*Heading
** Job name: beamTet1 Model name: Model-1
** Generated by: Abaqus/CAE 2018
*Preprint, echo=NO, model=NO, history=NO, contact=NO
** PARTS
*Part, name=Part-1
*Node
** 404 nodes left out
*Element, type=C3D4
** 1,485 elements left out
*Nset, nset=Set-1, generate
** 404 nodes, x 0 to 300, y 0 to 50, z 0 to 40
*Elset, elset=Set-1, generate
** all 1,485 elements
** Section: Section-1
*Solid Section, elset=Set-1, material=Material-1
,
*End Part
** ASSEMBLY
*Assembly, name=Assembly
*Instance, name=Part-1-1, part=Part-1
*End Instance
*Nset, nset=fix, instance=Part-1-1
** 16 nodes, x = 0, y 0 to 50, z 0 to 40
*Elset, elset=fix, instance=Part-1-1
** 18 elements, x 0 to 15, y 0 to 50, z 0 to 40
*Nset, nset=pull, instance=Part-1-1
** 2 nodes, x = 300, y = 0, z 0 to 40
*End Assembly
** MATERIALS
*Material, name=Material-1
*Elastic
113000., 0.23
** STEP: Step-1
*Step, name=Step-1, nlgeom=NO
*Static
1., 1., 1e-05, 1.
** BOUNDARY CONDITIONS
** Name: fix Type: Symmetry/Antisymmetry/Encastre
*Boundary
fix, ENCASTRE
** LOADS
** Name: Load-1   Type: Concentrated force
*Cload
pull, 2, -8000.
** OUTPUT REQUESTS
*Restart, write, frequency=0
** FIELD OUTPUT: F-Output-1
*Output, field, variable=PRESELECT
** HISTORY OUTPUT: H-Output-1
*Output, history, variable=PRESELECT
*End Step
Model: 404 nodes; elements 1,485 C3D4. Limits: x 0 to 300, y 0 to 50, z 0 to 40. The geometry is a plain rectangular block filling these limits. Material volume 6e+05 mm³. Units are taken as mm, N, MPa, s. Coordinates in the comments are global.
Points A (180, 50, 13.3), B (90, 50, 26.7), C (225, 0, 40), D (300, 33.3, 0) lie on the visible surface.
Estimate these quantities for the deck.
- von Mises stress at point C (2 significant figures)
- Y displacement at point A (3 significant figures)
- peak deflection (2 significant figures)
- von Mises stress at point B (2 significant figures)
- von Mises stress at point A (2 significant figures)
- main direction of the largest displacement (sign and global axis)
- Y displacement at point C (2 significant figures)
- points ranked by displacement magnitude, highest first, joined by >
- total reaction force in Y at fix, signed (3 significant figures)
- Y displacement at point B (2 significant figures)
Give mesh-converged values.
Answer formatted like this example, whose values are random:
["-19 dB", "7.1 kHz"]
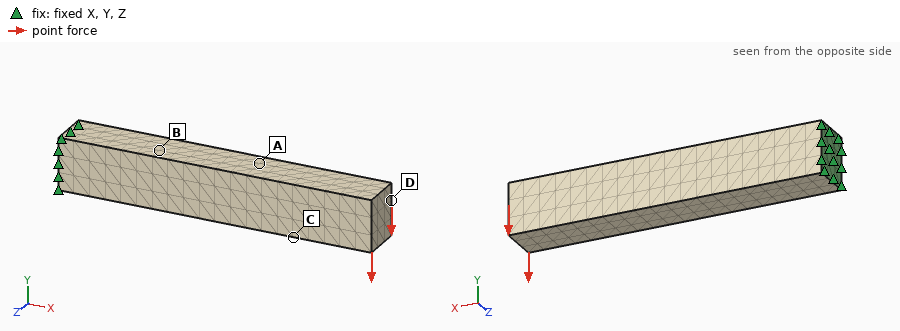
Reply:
["72 MPa", "-1.35 mm", "3.2 mm", "200 MPa", "120 MPa", "-Y", "-2.0 mm", "D > C > A > B", "16000 N", "-0.39 mm"]
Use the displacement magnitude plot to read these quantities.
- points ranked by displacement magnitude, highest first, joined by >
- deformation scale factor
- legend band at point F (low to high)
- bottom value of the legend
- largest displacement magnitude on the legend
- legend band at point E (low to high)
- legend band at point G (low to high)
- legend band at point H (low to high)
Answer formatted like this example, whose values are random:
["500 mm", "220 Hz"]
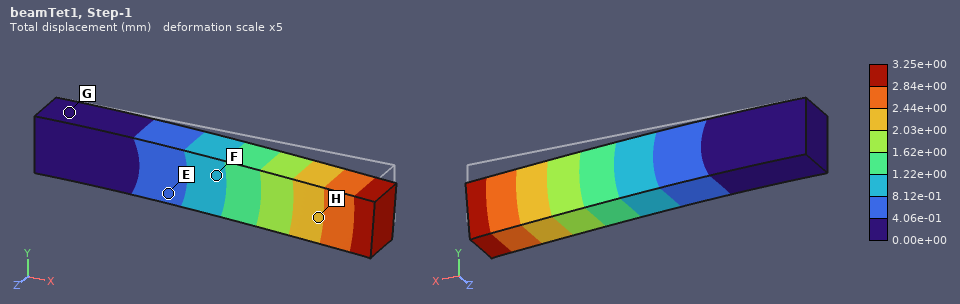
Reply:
["H > F > E > G", "5", "8.12e-01 to 1.22e+00 mm", "0.00e+00 mm", "3.25e+00 mm", "4.06e-01 to 8.12e-01 mm", "0.00e+00 to 4.06e-01 mm", "2.03e+00 to 2.44e+00 mm"]
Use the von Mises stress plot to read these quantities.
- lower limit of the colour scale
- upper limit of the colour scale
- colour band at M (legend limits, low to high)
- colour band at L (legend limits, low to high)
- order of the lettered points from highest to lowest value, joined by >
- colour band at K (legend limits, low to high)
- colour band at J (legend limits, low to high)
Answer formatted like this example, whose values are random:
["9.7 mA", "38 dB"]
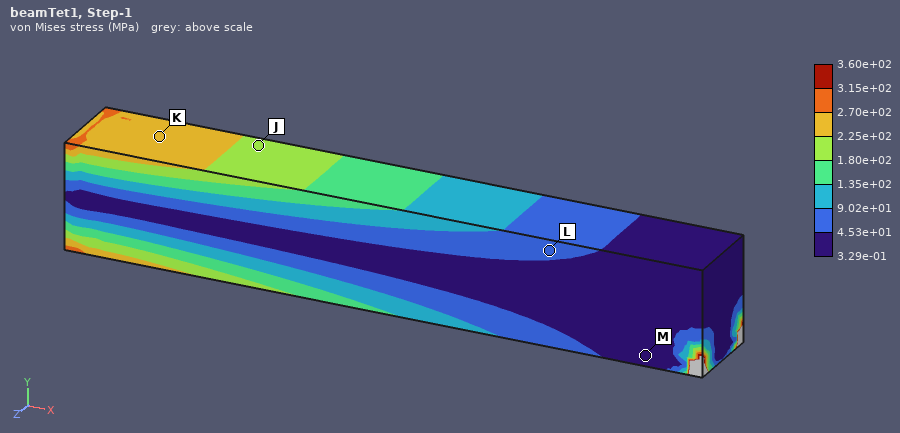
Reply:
["3.29e-01 MPa", "3.60e+02 MPa", "3.29e-01 to 4.53e+01 MPa", "4.53e+01 to 9.02e+01 MPa", "K > J > L > M", "2.25e+02 to 2.70e+02 MPa", "1.80e+02 to 2.25e+02 MPa"]
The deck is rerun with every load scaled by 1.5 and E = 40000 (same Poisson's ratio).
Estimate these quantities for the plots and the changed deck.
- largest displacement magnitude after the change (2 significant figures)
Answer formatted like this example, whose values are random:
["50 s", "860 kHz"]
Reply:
["14 mm"]
